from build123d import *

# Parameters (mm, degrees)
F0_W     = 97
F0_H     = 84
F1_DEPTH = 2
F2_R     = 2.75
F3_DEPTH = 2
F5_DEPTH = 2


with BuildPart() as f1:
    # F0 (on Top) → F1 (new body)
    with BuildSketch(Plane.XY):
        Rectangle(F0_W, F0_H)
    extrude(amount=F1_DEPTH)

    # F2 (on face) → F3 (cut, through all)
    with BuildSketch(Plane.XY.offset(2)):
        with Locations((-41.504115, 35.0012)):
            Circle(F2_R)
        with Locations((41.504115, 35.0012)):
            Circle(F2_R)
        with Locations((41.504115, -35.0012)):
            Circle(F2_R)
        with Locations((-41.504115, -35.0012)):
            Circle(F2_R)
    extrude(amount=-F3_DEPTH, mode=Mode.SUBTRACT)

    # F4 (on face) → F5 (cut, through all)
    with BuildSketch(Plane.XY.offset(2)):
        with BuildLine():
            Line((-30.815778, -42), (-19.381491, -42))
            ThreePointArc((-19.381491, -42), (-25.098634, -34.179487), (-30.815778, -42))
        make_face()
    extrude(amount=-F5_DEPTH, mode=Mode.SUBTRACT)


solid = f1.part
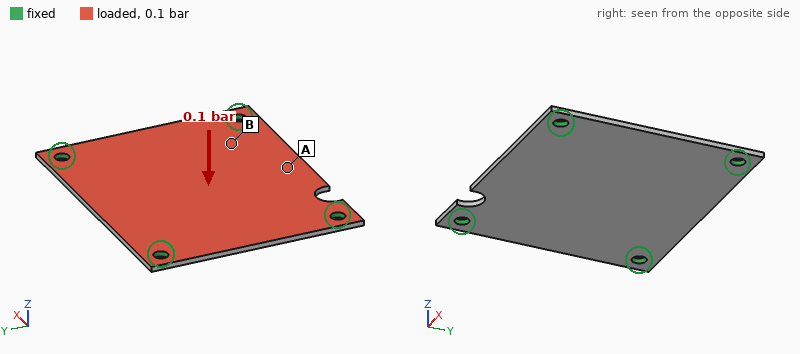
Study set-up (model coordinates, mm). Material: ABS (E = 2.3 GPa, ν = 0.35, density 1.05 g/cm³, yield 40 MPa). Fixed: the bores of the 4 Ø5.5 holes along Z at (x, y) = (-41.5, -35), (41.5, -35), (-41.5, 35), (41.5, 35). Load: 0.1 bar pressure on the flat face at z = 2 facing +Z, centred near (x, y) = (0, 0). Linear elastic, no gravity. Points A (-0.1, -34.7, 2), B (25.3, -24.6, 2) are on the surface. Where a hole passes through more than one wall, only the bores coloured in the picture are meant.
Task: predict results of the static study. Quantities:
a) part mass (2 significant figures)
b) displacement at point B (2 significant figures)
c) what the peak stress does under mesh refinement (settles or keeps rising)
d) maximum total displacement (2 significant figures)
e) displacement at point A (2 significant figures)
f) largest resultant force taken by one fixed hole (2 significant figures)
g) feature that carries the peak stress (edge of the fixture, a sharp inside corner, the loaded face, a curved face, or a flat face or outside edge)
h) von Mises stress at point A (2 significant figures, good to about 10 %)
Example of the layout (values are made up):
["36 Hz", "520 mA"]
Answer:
["17 g", "0.58 mm", "keeps rising", "1.4 mm", "1.00 mm", "20 N", "edge of the fixture", "5.1 MPa"]
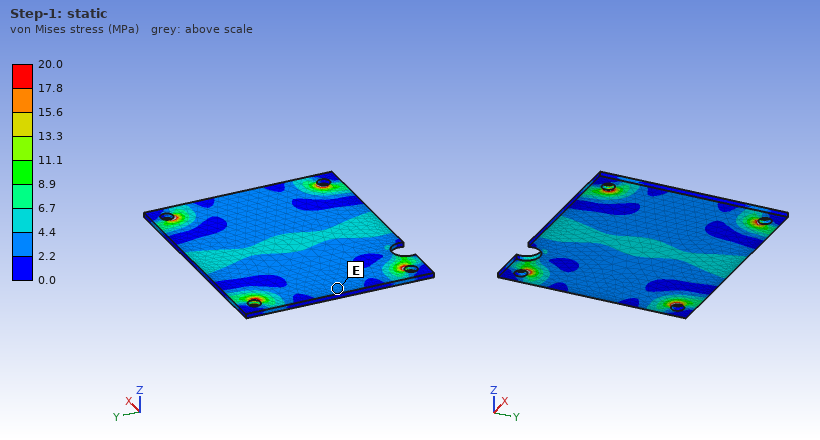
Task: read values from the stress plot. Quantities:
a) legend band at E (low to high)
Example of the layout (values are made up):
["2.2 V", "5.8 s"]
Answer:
["2.2 to 4.4 MPa"]
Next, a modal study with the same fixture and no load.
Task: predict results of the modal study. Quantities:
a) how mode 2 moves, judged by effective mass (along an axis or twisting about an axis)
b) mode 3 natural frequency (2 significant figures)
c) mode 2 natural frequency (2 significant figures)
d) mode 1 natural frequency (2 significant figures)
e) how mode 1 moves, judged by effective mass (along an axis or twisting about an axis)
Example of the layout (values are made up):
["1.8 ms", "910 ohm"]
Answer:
["twisting about X", "680 Hz", "540 Hz", "360 Hz", "along Z"]
